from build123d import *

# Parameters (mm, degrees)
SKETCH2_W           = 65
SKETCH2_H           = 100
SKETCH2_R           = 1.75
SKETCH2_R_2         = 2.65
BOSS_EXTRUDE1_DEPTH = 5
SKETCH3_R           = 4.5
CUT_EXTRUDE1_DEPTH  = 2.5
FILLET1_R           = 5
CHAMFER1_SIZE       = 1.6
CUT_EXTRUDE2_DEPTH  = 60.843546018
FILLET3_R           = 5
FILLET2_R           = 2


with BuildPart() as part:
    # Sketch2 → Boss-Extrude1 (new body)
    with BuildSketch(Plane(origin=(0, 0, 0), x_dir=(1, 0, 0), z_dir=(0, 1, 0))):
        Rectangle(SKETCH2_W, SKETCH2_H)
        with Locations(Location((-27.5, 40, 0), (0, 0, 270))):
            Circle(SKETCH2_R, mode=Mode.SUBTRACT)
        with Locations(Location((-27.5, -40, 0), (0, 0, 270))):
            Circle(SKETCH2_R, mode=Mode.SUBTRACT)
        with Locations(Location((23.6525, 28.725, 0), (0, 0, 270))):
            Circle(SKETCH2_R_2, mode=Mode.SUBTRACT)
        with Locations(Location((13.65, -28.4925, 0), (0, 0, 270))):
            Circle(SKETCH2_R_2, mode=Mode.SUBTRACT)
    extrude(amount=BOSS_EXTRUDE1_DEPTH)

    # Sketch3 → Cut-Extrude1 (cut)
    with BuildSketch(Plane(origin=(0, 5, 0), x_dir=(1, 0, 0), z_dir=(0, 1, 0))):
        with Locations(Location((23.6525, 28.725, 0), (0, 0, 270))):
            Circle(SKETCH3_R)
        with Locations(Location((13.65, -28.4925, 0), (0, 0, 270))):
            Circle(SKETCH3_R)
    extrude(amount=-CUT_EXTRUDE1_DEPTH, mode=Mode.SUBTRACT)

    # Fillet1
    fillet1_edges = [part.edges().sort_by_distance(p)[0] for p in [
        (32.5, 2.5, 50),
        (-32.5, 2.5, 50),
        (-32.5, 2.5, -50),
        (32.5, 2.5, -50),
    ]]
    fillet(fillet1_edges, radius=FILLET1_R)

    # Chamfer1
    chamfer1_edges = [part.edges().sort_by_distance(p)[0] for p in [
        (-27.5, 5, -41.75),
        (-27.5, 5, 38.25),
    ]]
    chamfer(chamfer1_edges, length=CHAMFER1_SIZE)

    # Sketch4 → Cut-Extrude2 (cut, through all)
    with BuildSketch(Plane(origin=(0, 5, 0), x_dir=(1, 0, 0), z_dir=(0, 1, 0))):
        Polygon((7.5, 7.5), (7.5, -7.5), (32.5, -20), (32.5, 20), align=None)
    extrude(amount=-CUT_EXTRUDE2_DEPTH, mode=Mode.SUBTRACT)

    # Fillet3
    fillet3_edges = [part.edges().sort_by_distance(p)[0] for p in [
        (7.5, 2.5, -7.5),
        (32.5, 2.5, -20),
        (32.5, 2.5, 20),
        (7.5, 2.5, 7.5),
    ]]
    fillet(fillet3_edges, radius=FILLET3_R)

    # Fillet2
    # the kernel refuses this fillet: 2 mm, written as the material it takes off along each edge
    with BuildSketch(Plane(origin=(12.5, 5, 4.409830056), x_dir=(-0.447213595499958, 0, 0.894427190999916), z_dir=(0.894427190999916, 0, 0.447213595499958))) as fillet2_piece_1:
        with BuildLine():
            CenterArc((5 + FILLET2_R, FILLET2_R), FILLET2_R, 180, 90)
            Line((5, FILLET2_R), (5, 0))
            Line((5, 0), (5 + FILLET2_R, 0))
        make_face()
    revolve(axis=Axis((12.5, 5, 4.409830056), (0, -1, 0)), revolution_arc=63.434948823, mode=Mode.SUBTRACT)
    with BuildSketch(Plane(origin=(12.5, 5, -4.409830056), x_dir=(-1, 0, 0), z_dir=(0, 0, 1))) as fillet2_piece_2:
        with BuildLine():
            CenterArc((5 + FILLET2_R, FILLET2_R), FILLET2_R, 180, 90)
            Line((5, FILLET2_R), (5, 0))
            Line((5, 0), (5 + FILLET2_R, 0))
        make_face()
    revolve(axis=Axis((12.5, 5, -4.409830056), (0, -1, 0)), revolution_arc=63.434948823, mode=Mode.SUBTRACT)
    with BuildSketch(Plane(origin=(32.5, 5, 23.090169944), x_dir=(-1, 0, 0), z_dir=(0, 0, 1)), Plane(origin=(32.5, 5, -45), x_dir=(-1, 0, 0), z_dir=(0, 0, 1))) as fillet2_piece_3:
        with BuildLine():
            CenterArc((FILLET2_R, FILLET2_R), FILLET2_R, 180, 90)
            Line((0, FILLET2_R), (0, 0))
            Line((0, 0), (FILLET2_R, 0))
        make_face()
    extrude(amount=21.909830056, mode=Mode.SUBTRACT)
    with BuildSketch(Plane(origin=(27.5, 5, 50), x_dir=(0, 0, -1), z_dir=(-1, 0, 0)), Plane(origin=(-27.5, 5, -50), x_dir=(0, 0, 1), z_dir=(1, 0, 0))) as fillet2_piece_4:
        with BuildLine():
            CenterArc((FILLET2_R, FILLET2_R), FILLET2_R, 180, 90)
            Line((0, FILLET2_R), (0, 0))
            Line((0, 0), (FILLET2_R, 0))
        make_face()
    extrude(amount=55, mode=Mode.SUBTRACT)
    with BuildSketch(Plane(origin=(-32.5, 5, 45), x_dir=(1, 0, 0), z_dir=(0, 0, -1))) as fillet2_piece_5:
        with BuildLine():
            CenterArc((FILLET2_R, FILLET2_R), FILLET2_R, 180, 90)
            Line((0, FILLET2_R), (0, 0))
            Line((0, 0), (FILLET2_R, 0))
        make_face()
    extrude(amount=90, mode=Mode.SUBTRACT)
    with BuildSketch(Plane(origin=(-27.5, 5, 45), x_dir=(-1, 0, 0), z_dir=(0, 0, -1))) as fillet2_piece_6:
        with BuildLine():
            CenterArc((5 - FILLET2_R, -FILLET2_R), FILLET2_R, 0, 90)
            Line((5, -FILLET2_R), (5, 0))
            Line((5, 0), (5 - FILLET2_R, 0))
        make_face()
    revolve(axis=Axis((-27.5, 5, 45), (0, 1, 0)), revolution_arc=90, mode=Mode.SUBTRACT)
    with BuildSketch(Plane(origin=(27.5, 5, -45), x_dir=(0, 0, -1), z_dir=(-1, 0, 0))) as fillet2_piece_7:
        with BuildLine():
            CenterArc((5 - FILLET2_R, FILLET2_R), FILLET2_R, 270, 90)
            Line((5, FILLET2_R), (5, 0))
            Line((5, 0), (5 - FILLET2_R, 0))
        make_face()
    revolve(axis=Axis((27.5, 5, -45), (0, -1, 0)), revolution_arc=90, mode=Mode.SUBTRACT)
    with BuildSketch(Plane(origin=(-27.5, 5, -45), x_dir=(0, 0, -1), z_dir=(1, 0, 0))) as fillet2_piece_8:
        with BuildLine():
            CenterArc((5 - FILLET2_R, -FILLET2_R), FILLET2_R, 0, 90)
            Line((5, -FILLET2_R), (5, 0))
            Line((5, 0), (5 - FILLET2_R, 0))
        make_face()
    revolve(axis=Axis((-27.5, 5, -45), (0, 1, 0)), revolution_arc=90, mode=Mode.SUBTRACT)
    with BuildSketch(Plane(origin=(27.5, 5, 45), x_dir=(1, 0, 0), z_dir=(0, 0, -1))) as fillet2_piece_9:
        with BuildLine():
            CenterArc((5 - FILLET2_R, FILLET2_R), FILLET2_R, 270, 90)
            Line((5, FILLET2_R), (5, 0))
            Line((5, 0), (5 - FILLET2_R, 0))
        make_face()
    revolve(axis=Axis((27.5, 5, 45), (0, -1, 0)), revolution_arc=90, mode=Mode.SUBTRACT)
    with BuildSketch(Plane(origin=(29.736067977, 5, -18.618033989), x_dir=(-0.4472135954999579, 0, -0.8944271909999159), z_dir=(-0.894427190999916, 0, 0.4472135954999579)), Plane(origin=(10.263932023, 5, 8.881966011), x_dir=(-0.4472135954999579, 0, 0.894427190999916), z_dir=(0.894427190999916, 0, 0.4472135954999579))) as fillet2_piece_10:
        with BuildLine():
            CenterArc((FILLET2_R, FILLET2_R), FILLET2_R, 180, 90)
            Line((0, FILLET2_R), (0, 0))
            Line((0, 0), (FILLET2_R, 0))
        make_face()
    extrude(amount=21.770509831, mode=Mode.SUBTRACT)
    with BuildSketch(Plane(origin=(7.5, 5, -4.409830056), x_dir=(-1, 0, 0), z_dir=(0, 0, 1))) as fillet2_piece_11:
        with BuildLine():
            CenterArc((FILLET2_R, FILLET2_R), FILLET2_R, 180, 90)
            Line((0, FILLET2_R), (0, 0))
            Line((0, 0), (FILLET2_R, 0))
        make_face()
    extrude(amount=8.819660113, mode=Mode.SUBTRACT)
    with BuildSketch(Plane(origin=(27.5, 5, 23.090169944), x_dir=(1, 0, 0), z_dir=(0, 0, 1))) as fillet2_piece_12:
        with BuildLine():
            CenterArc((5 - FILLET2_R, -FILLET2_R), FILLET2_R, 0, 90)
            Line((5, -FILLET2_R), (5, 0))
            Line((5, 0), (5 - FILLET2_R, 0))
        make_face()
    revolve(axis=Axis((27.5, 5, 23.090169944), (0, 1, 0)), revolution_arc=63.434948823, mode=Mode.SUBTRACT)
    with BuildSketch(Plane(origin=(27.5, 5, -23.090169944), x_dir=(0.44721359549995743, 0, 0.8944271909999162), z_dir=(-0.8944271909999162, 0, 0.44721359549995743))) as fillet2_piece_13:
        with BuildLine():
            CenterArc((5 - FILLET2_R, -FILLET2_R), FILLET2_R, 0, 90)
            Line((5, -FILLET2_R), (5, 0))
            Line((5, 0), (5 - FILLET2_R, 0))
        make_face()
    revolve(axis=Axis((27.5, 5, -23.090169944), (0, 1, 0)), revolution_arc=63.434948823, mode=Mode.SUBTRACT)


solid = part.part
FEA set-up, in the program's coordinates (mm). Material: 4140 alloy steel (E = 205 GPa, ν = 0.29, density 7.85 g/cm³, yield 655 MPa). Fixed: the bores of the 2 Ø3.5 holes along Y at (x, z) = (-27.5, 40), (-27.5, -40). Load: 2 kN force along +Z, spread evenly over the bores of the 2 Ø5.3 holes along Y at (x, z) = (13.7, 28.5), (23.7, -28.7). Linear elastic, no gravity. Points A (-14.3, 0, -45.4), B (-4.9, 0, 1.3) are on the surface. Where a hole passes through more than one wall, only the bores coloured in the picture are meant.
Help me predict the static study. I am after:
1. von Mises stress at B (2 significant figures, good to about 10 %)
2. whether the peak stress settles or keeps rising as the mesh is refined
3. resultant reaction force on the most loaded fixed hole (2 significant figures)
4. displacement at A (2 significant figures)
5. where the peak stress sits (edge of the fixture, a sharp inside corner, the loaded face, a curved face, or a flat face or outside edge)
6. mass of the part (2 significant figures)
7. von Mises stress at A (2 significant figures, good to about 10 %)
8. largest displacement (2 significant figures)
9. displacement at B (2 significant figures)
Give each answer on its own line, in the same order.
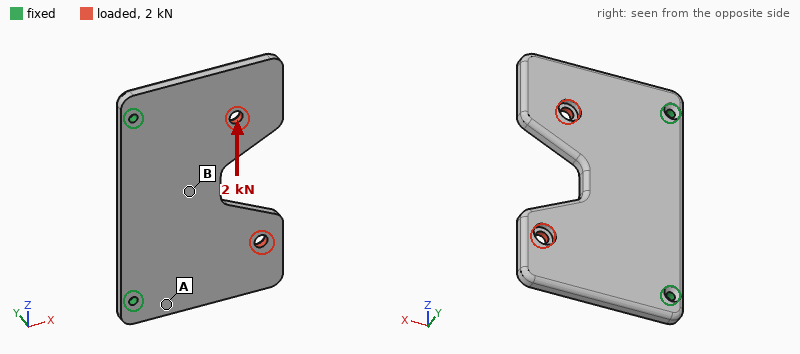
17 MPa
keeps rising
1.6 kN
3.5 µm
edge of the fixture
220 g
7.8 MPa
18 µm
3.3 µm
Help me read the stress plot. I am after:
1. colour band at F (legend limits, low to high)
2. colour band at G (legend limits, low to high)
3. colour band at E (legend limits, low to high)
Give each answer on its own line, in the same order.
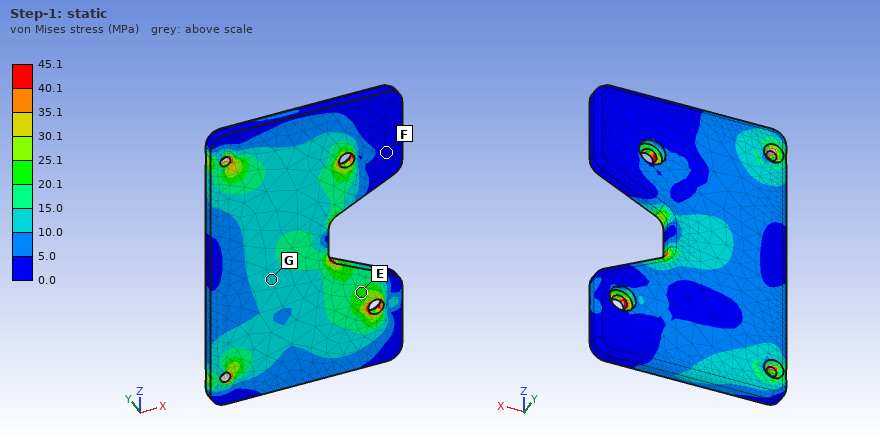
0.0 to 5.0 MPa
10.0 to 15.0 MPa
20.1 to 25.1 MPa
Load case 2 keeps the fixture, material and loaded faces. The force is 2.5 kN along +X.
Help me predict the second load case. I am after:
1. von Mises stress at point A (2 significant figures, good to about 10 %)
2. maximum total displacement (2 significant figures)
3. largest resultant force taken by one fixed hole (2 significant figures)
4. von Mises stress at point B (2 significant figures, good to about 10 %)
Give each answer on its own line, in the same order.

20 MPa
42 µm
1.3 kN
5.5 MPa
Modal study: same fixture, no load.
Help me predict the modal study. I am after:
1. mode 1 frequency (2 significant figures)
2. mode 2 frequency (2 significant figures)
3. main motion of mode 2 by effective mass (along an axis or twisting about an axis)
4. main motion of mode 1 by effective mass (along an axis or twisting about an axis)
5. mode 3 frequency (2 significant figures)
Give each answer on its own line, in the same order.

870 Hz
1500 Hz
twisting about X
along Y
2800 Hz
